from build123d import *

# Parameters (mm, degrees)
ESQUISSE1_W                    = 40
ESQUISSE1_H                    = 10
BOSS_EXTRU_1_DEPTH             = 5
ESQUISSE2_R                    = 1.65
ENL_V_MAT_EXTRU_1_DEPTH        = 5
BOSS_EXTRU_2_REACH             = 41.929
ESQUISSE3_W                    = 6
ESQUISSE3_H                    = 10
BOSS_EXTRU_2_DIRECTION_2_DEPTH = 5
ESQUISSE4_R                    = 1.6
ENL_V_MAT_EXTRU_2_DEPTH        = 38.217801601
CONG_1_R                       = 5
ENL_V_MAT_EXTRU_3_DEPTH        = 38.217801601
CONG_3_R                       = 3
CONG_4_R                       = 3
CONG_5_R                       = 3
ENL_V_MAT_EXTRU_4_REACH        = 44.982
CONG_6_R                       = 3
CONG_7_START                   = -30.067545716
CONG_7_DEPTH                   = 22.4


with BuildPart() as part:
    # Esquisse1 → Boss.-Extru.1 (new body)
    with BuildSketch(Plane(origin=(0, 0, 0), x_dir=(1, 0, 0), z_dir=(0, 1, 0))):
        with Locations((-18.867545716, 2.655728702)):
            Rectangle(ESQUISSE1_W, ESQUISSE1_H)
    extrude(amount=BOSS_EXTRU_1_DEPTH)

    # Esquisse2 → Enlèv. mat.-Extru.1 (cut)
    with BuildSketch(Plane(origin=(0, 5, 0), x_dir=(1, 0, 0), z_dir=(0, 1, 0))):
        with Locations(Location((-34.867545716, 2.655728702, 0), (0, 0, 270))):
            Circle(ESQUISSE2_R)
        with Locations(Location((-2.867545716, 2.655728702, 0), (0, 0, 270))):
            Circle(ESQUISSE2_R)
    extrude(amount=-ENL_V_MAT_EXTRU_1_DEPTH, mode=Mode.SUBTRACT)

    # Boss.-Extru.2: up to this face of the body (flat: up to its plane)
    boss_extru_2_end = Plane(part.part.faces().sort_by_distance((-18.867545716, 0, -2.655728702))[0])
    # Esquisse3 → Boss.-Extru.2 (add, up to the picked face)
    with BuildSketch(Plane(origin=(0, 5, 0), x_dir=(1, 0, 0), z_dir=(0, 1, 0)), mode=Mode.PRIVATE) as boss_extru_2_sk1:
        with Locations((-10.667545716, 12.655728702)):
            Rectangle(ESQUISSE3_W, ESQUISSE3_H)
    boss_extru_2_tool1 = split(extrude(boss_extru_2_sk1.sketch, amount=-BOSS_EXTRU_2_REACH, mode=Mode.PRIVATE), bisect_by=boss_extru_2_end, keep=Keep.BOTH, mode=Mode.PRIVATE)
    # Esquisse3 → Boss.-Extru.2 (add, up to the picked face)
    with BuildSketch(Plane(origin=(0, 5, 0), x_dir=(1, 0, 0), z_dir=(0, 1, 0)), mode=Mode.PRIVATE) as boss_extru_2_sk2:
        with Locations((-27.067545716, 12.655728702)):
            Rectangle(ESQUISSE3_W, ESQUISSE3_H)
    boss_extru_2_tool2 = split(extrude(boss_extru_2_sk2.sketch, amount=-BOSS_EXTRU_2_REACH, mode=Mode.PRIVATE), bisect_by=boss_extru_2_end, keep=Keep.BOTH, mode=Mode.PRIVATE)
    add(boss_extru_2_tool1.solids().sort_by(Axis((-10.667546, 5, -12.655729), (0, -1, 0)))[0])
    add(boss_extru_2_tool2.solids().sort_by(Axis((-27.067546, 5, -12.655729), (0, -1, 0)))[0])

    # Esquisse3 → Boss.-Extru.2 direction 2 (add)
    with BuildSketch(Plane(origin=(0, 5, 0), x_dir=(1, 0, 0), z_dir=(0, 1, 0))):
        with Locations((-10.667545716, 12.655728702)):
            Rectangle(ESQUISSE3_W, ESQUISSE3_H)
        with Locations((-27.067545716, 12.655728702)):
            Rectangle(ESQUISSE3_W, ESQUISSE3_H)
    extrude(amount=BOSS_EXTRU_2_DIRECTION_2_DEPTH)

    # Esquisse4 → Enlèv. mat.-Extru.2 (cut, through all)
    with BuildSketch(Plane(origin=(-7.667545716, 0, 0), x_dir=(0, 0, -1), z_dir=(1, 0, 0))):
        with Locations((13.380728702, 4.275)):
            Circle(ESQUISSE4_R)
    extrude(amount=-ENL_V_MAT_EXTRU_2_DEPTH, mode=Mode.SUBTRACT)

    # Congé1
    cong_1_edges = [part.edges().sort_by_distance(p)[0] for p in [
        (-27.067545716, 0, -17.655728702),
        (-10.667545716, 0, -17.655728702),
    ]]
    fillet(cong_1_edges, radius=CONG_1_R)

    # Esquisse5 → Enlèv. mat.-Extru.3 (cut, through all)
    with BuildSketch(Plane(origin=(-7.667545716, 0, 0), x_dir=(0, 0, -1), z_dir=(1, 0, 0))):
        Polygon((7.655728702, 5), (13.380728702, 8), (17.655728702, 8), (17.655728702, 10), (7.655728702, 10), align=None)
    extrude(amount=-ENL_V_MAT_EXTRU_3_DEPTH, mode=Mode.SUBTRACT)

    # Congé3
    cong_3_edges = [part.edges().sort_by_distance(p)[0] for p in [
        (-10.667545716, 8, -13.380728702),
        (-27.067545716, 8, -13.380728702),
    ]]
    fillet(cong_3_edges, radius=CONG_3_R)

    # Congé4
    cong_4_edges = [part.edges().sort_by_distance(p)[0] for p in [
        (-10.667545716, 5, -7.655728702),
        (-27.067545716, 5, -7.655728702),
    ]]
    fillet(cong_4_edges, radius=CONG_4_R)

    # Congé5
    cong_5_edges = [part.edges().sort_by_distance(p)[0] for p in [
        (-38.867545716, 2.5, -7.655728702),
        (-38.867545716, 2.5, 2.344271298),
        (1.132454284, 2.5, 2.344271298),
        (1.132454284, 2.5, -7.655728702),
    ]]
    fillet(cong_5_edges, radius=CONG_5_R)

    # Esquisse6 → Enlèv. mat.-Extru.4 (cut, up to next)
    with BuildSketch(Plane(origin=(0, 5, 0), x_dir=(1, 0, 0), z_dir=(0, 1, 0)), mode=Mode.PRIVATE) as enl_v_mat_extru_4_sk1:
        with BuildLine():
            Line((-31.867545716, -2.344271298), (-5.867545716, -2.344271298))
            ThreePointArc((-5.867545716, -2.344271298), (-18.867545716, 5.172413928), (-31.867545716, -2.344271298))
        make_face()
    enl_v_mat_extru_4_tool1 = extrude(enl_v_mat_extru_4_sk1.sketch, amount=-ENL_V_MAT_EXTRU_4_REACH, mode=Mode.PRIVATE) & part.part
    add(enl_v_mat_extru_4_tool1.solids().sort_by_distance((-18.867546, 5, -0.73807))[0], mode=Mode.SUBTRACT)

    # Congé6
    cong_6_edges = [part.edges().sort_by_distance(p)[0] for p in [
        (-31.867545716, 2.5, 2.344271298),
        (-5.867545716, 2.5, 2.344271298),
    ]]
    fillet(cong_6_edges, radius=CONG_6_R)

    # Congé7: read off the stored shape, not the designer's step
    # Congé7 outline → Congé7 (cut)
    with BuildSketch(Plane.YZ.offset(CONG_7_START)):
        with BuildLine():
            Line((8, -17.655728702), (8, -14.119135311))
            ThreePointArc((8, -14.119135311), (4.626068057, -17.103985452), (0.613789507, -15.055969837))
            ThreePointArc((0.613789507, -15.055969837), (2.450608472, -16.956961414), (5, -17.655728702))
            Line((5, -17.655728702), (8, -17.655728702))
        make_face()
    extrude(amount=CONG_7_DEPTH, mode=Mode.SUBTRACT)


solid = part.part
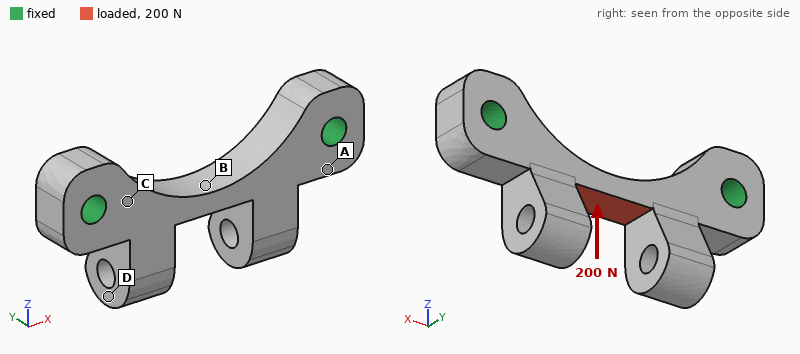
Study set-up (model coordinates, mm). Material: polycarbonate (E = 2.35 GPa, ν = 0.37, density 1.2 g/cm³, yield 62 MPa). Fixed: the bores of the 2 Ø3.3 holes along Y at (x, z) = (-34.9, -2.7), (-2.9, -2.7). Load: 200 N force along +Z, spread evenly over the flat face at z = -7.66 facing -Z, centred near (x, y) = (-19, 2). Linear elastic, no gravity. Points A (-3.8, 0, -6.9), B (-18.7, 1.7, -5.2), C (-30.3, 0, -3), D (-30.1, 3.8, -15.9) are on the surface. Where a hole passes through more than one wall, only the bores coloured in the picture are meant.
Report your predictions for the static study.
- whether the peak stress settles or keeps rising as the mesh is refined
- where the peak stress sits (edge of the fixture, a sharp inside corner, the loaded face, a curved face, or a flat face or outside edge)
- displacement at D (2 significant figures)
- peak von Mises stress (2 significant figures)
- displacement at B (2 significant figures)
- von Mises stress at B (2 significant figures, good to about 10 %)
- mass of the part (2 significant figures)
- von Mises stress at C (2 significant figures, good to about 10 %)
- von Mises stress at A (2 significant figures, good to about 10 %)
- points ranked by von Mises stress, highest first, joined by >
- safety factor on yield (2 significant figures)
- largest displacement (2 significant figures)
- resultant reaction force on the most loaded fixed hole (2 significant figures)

settles
the loaded face
0.19 mm
32 MPa
0.24 mm
14 MPa
2.2 g
10 MPa
5.2 MPa
B > C > A > D
1.9
0.25 mm
160 N
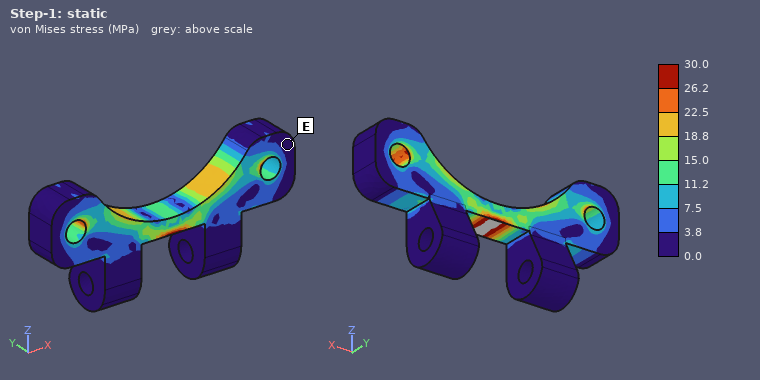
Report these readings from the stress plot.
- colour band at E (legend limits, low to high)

0.0 to 3.8 MPa
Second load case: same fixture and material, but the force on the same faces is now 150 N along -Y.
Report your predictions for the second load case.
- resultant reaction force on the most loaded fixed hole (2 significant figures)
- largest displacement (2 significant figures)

75 N
0.30 mm
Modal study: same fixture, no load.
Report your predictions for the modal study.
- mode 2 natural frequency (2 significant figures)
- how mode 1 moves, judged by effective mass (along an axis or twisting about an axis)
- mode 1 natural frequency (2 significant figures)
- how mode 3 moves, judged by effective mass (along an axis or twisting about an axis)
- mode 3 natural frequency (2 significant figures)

4100 Hz
along Y
3600 Hz
along Z
5100 Hz
